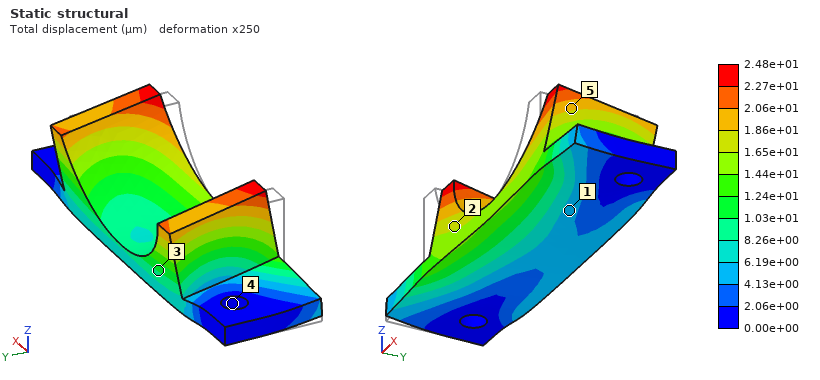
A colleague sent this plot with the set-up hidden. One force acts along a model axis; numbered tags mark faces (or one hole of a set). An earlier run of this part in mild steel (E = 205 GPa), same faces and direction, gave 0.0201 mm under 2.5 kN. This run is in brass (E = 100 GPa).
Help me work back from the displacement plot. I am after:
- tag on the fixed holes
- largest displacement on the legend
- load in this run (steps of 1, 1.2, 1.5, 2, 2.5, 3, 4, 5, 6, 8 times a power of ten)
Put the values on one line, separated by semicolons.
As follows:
4; 2.48e+01 µm; 1.5 kN
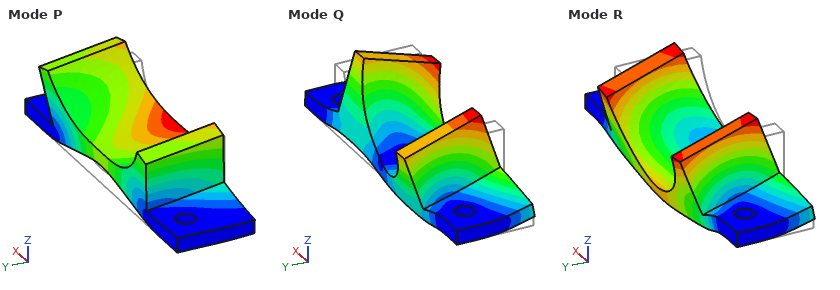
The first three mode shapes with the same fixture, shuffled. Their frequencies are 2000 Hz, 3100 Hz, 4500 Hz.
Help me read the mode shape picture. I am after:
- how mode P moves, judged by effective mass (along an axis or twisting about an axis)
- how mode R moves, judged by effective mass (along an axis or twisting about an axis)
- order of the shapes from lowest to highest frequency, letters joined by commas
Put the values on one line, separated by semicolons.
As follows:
along Z; along Y; P, R, Q
